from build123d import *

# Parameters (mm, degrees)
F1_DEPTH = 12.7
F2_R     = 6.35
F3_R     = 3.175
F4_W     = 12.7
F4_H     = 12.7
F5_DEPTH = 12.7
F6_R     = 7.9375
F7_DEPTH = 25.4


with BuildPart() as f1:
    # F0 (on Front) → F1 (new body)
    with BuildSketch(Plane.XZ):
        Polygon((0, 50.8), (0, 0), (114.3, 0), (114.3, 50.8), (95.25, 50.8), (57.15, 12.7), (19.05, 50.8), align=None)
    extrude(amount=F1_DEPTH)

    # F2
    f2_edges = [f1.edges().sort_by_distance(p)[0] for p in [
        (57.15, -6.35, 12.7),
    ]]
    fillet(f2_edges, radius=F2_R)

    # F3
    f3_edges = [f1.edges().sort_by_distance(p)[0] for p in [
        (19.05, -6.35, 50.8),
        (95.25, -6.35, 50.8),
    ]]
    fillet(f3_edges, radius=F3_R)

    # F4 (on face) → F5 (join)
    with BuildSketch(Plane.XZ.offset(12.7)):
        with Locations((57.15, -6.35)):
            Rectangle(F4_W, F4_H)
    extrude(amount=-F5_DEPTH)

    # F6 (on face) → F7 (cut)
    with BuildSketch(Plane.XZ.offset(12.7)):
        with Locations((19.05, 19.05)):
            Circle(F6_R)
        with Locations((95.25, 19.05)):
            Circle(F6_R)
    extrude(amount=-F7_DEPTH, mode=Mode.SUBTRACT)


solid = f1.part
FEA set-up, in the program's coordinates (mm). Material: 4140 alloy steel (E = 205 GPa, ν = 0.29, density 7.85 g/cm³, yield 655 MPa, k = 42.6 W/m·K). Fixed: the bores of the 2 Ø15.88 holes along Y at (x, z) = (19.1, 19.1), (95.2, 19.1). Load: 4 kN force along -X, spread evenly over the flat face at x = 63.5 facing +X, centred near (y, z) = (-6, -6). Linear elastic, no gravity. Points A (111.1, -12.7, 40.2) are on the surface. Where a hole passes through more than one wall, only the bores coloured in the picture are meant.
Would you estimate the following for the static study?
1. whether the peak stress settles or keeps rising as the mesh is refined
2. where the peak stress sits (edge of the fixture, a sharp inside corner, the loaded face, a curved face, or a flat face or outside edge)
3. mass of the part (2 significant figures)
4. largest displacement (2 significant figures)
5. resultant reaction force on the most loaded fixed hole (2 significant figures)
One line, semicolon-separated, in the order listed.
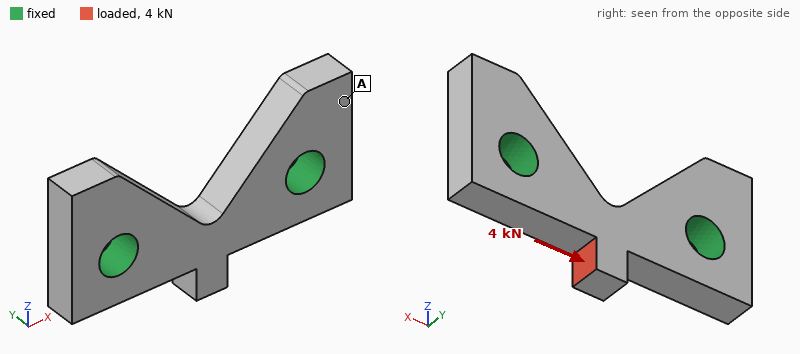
keeps rising; a sharp inside corner; 410 g; 13 µm; 2.6 kN
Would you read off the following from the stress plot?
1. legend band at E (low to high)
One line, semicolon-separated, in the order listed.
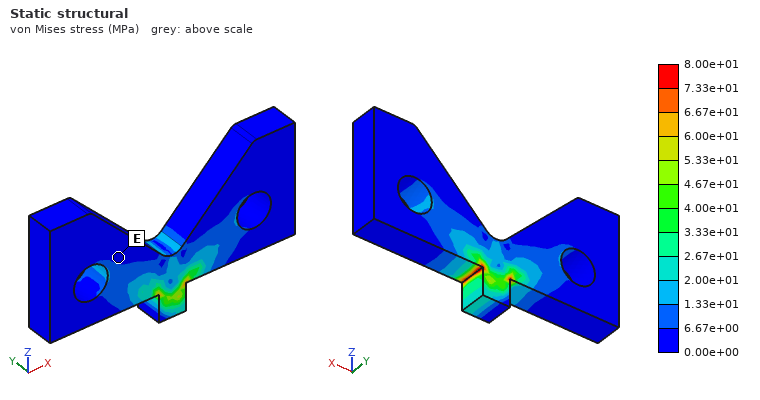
0.00e+00 to 6.67e+00 MPa
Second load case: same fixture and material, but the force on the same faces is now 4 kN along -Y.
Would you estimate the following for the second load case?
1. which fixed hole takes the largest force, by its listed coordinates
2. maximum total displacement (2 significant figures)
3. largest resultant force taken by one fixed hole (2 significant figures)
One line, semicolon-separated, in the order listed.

(95.2, 19.1); 61 µm; 2.5 kN
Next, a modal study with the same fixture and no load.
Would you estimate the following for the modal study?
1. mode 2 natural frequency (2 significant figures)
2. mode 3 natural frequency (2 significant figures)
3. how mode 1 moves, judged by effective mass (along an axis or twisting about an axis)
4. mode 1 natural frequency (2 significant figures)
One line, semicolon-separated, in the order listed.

14 kHz; 14 kHz; along Y; 9500 Hz
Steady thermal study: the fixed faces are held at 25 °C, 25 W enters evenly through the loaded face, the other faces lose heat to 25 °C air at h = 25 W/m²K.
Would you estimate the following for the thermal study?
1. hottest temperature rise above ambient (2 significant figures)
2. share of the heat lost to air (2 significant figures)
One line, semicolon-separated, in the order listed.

77 K; 9.9 %
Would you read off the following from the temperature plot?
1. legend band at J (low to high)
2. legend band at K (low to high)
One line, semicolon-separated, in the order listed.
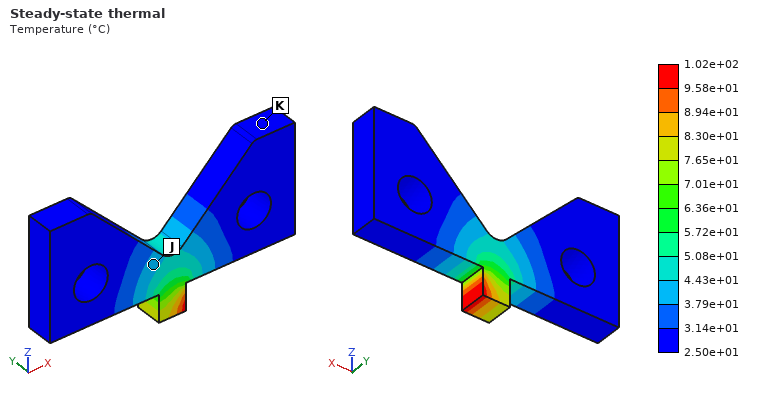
3.79e+01 to 4.43e+01 °C; 2.50e+01 to 3.14e+01 °C
